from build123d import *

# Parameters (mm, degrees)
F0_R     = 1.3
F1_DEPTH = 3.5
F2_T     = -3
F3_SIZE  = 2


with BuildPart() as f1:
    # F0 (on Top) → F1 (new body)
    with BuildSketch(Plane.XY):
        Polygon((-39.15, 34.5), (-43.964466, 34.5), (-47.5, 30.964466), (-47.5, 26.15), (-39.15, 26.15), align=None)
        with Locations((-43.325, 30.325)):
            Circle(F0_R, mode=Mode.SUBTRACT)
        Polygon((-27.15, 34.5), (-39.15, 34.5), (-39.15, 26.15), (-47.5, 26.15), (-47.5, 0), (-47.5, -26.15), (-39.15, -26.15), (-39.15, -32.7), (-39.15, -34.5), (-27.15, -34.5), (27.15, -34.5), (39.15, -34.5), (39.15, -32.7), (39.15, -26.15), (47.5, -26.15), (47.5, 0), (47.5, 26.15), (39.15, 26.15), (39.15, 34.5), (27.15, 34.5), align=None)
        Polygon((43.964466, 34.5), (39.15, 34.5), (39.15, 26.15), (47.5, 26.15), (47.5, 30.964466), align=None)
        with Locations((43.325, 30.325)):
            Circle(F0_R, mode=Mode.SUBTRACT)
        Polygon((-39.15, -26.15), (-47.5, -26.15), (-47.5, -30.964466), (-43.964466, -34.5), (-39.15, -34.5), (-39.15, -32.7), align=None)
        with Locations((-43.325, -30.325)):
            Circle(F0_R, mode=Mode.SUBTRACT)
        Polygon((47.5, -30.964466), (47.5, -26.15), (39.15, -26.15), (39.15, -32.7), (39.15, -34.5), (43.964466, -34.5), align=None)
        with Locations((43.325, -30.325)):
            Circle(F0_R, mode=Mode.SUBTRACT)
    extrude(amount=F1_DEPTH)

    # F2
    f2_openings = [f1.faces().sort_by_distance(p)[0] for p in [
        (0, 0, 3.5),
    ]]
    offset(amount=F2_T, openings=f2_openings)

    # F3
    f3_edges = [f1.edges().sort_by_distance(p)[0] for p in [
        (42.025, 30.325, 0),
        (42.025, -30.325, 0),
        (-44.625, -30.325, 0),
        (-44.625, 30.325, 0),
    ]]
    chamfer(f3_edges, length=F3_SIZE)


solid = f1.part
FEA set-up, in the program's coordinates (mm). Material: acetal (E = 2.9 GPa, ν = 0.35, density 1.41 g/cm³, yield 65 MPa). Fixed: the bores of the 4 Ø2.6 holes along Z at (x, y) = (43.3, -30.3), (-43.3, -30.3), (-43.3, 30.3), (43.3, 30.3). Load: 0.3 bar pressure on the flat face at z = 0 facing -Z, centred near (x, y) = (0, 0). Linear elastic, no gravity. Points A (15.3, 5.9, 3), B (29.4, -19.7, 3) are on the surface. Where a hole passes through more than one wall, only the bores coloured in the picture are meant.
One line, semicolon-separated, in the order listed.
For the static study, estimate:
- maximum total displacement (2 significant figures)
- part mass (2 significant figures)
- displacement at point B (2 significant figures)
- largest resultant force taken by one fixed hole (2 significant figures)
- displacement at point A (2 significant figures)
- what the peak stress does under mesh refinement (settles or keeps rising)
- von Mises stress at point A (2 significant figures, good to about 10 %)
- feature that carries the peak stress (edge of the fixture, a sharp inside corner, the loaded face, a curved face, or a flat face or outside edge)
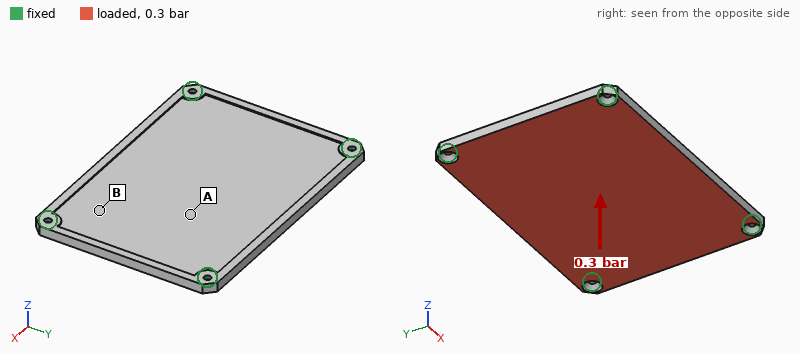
1.3 mm; 28 g; 0.60 mm; 130 N; 1.2 mm; keeps rising; 5.6 MPa; edge of the fixture
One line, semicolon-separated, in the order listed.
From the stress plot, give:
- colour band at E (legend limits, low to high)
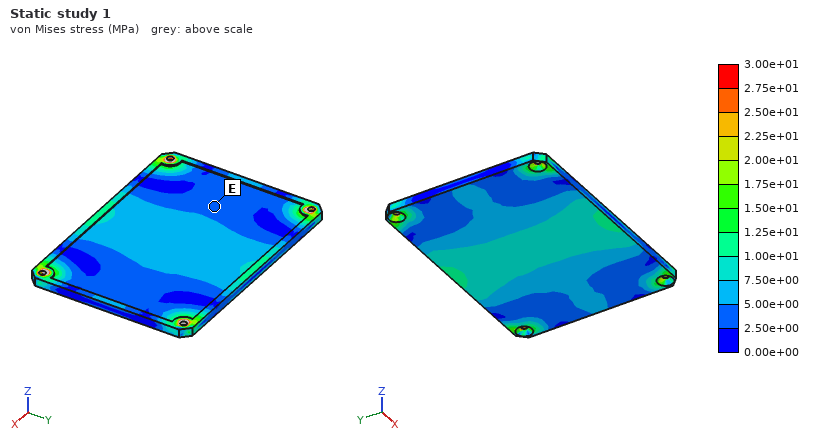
2.50e+00 to 5.00e+00 MPa
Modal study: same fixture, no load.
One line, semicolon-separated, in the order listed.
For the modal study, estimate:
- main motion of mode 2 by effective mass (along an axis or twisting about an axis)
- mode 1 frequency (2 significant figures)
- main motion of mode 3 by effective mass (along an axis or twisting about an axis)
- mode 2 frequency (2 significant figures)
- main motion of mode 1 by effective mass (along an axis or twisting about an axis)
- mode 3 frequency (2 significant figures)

twisting about X; 420 Hz; twisting about Y; 700 Hz; along Z; 980 Hz
